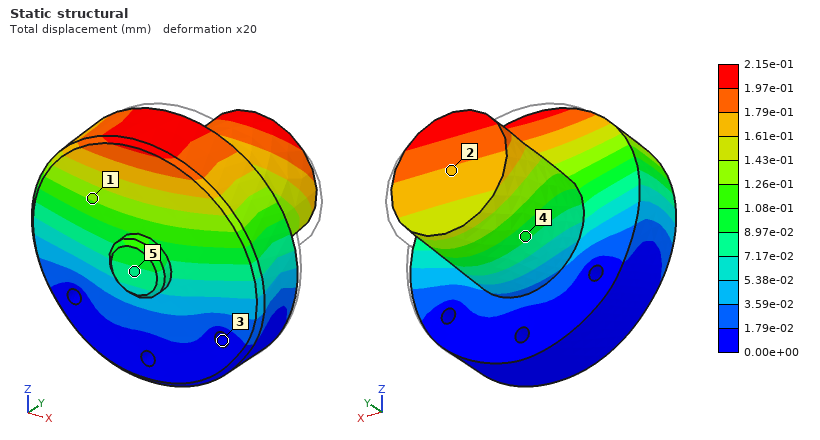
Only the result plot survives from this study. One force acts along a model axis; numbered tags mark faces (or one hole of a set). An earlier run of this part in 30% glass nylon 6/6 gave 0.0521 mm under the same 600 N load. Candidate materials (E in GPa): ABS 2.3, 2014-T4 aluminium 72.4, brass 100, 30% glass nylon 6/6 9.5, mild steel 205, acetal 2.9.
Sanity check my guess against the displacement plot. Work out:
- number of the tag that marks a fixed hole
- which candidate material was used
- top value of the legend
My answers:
3
ABS
2.15e-01 mm
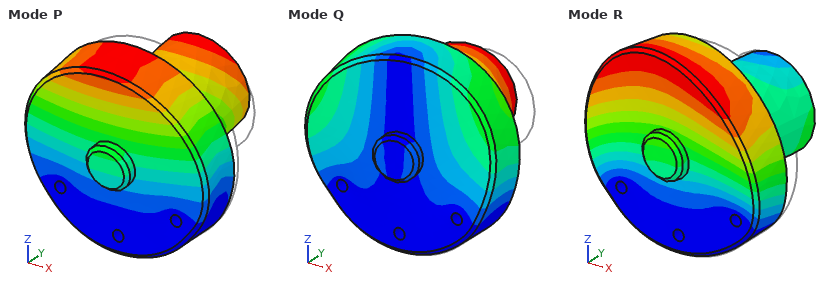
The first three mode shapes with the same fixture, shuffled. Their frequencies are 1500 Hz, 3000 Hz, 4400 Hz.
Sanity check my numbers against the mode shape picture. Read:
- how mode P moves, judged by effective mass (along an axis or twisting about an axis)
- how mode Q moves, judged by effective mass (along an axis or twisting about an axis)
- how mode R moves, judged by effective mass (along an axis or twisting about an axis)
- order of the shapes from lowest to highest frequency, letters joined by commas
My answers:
along Y
along X
along X
P, Q, R
